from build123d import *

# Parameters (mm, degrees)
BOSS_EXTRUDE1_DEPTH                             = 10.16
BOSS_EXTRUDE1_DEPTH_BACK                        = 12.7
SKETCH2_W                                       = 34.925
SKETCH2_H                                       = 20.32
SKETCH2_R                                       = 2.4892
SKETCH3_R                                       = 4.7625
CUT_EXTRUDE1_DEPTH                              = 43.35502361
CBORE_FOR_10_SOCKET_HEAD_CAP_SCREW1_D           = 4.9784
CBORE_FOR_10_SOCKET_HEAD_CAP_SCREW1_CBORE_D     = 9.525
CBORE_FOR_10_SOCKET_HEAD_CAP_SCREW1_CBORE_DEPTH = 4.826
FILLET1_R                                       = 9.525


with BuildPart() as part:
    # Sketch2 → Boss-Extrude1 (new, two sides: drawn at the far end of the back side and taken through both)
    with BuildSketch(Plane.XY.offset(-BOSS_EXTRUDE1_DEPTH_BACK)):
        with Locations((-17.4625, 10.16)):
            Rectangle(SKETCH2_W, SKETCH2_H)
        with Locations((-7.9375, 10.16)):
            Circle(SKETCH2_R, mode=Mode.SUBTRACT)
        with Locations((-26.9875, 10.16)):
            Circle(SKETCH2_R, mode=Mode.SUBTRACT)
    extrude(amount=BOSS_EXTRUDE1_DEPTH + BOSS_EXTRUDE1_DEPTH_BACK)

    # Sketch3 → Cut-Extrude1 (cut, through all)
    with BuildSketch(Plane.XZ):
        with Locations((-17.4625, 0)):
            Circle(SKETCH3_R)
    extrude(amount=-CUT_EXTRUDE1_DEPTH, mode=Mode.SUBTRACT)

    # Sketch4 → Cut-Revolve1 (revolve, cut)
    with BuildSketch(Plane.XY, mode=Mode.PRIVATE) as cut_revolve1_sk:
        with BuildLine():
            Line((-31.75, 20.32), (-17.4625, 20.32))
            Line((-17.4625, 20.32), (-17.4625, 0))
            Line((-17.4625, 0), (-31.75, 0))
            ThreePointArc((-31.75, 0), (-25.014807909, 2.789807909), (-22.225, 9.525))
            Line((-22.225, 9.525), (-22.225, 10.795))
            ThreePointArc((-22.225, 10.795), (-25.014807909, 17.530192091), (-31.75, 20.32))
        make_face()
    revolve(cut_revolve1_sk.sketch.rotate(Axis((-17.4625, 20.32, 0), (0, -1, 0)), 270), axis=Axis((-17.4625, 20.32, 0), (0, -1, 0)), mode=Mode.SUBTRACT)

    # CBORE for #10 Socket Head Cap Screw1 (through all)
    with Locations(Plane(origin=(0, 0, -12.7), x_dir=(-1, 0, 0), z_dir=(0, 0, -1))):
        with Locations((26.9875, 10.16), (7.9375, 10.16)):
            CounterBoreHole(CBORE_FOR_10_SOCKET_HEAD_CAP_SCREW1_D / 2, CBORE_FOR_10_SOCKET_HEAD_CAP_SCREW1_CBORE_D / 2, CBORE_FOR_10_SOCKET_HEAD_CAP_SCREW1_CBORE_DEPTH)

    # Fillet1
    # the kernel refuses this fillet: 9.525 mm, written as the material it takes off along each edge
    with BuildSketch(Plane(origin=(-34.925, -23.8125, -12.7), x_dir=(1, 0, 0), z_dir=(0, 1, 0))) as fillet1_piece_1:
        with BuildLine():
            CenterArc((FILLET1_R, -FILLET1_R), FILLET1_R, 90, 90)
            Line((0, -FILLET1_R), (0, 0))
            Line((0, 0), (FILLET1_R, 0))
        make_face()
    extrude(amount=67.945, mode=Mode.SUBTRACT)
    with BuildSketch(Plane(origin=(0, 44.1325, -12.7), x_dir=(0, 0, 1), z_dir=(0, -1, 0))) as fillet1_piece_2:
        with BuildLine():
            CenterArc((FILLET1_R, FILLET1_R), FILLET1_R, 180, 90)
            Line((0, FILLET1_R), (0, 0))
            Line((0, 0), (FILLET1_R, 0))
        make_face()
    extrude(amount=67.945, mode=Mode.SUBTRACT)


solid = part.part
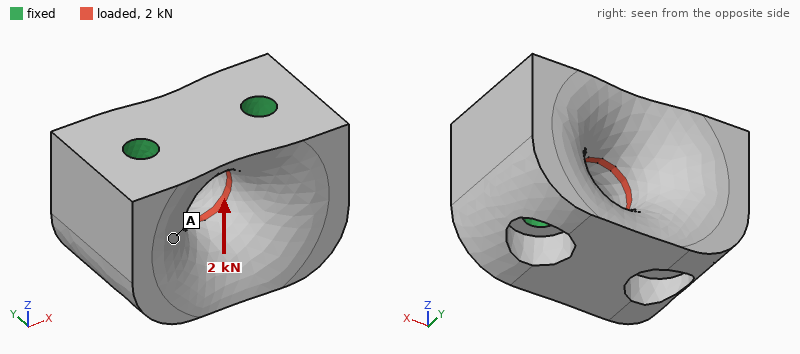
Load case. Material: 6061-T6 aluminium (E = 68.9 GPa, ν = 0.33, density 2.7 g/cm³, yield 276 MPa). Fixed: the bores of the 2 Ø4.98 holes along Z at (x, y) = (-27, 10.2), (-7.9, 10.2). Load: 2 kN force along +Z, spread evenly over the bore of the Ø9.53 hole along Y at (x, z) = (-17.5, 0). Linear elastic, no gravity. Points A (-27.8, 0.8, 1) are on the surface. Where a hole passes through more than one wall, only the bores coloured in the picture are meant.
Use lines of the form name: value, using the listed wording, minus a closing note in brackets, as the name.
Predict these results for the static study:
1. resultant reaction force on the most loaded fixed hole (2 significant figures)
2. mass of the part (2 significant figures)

resultant reaction force on the most loaded fixed hole: 1.0 kN
mass of the part: 30 g
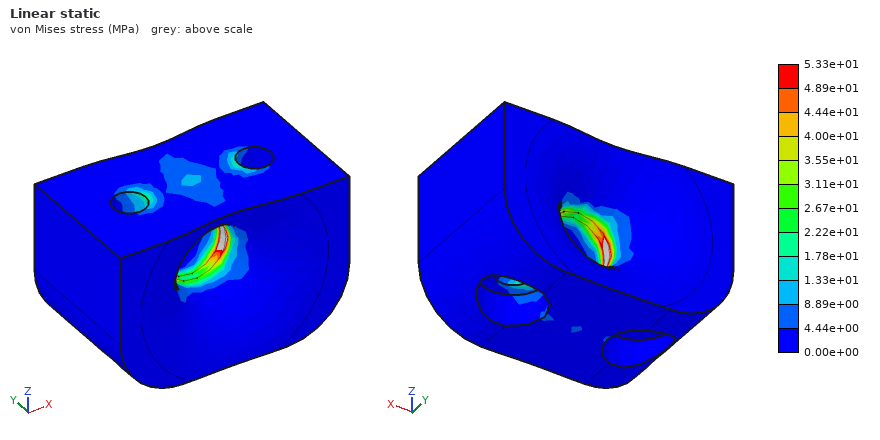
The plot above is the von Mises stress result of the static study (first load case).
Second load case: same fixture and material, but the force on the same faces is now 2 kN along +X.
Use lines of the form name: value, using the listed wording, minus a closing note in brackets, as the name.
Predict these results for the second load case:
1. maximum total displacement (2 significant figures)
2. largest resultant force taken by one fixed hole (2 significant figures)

maximum total displacement: 1.8 µm
largest resultant force taken by one fixed hole: 1.0 kN
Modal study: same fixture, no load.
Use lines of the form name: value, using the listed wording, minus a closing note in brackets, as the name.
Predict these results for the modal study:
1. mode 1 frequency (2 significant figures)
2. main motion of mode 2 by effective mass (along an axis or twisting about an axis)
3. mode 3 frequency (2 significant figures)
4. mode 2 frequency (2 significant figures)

mode 1 frequency: 40 kHz
main motion of mode 2 by effective mass: twisting about Z
mode 3 frequency: 52 kHz
mode 2 frequency: 50 kHz
